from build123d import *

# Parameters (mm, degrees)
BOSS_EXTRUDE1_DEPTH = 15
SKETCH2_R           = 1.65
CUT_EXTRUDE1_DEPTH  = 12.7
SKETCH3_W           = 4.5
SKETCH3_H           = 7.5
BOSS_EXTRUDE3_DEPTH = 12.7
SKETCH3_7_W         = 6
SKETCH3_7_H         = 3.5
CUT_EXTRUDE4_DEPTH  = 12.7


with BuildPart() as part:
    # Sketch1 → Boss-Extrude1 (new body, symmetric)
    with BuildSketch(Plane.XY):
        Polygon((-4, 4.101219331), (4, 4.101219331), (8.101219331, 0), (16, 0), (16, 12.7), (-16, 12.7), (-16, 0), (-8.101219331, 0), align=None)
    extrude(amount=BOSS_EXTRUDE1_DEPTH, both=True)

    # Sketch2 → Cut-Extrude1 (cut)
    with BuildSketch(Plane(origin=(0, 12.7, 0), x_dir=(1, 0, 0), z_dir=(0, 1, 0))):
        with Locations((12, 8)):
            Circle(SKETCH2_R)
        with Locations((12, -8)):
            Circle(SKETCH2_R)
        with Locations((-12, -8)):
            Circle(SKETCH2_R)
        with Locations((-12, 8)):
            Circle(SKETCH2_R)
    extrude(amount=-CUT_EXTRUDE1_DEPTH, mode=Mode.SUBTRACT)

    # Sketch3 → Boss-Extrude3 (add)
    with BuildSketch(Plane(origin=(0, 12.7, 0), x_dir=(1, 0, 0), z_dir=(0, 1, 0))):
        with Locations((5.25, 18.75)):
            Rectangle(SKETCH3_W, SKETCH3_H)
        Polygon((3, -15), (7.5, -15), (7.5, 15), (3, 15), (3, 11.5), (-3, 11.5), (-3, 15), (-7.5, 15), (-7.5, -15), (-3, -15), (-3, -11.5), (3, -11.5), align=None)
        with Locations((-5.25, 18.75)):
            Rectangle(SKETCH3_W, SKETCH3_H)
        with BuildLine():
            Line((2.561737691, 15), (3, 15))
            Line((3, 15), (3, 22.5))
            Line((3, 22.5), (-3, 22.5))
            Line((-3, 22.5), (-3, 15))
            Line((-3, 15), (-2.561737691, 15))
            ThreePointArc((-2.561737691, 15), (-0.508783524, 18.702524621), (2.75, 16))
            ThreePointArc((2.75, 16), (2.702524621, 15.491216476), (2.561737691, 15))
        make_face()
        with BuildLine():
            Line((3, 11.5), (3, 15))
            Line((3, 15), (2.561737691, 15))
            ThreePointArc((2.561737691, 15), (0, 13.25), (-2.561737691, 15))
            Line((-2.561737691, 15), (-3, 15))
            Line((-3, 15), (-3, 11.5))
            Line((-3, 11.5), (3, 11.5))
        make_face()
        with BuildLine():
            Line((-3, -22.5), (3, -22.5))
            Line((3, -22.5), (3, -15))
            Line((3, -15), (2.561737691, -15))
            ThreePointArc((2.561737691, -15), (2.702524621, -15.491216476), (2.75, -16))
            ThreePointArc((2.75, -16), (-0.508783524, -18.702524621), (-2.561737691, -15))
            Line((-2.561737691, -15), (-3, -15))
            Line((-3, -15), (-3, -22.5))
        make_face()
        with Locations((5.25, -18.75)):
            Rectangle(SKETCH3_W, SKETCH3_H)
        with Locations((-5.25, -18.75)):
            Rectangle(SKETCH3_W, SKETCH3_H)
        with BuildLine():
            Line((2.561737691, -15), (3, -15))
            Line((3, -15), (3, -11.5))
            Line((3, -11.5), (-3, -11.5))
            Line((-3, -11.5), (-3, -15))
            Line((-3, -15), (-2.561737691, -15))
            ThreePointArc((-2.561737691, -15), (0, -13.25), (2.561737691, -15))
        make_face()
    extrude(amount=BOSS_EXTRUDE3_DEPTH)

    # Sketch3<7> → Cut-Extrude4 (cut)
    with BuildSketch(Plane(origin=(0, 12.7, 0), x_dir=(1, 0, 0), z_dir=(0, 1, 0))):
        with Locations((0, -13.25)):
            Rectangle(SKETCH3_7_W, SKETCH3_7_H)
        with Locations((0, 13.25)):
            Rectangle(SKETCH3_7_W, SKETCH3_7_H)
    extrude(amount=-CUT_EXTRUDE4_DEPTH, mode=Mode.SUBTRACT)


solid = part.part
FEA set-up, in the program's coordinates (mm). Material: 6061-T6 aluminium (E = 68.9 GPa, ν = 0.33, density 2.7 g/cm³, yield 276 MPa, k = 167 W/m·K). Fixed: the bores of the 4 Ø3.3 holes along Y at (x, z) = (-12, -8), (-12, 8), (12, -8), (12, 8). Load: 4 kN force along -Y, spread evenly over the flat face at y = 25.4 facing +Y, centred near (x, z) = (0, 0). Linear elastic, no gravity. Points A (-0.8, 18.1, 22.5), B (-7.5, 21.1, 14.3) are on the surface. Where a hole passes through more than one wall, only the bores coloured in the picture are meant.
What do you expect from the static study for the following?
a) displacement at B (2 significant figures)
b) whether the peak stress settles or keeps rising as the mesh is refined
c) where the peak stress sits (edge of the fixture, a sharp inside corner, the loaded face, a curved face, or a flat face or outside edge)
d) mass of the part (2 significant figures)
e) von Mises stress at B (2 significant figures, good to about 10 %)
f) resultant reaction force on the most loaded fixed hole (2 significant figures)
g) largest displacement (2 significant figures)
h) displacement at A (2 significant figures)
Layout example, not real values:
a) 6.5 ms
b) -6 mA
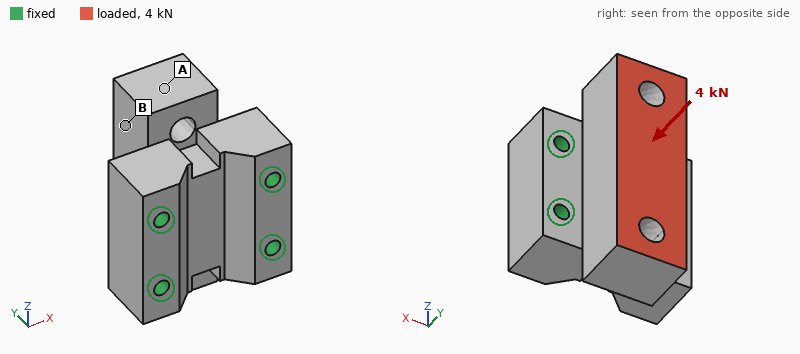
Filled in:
a) 4.5 µm
b) keeps rising
c) edge of the fixture
d) 48 g
e) 10 MPa
f) 1.1 kN
g) 7.6 µm
h) 6.7 µm
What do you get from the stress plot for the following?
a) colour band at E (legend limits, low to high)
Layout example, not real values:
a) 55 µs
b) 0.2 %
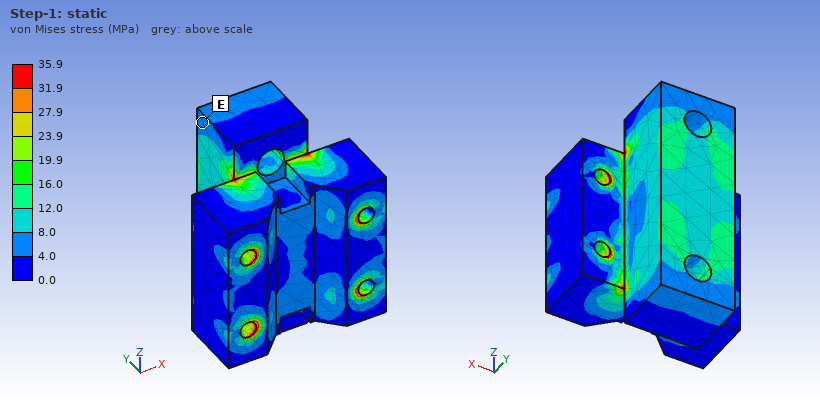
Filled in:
a) 4.0 to 8.0 MPa
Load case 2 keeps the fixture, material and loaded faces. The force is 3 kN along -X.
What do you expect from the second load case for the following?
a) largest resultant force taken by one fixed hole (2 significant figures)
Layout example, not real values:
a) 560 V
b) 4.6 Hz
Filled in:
a) 1.5 kN
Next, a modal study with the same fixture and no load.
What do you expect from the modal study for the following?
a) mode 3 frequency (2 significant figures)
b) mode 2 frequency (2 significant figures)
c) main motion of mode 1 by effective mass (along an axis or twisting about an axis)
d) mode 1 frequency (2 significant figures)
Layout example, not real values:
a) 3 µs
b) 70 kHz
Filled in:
a) 24 kHz
b) 24 kHz
c) along Z
d) 18 kHz
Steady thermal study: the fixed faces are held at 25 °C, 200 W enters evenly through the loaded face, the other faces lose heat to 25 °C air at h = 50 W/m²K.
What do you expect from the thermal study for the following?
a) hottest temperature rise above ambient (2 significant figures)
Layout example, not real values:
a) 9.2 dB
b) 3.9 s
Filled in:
a) 54 K
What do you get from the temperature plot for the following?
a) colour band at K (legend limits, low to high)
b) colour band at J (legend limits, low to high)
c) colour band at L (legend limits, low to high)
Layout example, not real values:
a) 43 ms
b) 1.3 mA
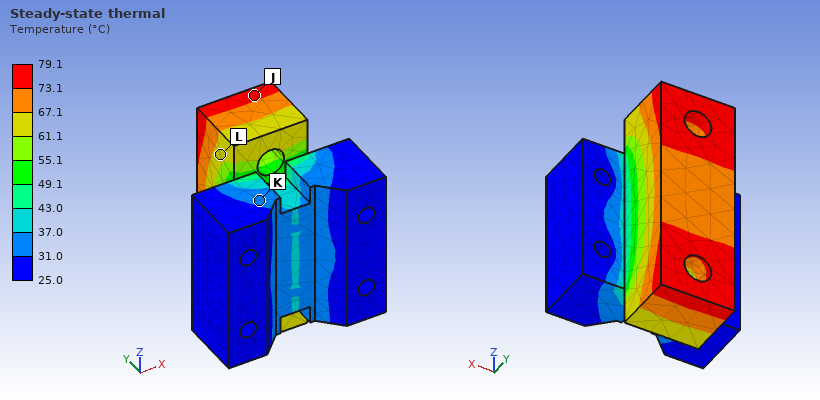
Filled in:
a) 31.0 to 37.0 °C
b) 73.1 to 79.1 °C
c) 61.1 to 67.1 °C
